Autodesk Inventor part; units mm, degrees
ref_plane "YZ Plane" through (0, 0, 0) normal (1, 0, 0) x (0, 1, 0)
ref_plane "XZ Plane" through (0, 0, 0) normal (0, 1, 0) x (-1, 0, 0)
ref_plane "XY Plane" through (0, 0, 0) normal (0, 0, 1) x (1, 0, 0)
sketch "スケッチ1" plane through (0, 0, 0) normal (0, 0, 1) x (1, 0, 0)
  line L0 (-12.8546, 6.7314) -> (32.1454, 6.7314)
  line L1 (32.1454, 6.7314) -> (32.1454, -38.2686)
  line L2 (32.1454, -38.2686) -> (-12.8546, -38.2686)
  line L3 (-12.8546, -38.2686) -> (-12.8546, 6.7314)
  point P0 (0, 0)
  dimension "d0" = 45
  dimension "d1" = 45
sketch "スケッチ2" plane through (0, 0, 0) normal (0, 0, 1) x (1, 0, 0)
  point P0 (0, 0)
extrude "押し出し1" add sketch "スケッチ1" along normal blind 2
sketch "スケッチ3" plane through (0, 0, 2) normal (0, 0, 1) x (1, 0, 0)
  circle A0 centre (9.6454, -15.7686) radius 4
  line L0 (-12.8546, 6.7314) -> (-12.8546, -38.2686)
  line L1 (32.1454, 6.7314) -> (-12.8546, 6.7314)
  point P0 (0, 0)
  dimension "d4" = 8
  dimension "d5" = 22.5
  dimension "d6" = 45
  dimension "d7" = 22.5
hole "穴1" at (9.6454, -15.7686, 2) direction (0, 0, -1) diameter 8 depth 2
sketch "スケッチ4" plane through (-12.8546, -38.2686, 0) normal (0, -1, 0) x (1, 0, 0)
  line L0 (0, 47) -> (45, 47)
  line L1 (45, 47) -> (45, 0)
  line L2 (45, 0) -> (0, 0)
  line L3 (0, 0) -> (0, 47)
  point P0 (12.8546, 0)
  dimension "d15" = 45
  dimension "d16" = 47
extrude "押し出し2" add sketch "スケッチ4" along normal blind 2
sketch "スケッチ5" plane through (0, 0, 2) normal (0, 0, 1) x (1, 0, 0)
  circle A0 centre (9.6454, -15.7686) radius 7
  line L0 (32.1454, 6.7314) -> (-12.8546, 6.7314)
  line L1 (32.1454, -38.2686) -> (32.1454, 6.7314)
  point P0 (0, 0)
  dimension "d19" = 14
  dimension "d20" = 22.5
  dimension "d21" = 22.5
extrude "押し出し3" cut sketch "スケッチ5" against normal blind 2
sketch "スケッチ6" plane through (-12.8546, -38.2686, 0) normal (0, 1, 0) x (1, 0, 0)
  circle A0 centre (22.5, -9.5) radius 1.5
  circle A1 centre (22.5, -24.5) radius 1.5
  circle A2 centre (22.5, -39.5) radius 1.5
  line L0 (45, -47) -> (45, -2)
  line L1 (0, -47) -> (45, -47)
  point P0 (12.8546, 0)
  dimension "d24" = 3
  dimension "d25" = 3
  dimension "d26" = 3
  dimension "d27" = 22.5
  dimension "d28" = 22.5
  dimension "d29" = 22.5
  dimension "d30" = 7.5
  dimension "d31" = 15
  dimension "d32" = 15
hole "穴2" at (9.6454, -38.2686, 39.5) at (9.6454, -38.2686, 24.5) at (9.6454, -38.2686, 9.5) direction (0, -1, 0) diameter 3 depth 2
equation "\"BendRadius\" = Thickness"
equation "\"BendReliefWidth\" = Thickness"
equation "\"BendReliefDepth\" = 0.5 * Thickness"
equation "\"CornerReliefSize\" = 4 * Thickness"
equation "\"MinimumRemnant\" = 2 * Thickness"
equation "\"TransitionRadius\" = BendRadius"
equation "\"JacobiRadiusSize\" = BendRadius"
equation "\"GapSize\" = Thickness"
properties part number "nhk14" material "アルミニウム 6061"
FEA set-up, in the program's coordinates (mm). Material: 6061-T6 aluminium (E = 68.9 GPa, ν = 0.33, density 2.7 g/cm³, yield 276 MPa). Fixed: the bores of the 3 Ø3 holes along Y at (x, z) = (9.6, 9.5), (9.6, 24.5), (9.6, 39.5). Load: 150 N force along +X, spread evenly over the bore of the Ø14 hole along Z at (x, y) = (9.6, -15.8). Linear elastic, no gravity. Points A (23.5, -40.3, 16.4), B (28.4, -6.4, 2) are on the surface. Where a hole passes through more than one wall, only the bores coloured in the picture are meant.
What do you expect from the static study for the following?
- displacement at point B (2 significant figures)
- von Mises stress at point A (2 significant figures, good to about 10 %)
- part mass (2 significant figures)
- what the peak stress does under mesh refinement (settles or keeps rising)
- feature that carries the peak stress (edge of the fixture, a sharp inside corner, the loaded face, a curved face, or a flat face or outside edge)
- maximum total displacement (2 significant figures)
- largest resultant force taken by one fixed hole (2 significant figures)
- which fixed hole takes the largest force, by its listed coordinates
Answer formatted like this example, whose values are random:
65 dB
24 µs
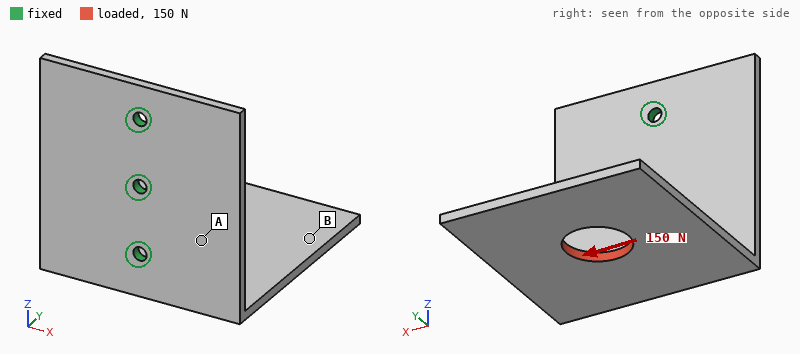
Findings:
0.42 mm
37 MPa
21 g
keeps rising
edge of the fixture
0.57 mm
180 N
(9.6, 9.5)
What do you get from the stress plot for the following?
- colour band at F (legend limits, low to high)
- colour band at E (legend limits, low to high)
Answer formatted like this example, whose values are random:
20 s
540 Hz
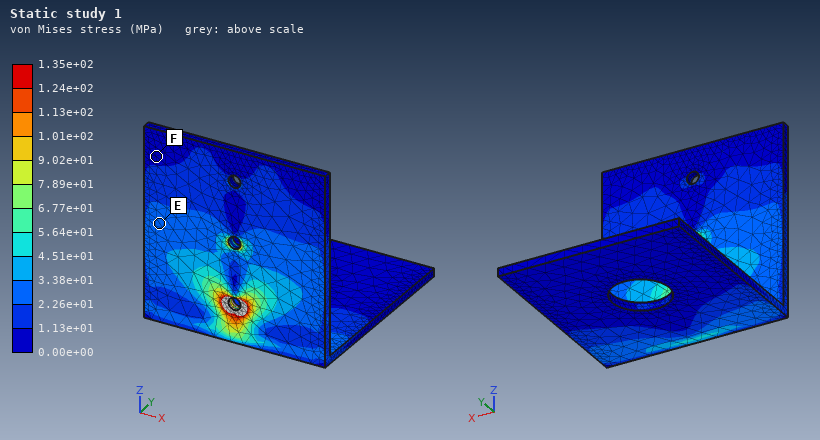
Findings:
0.00e+00 to 1.13e+01 MPa
2.26e+01 to 3.38e+01 MPa
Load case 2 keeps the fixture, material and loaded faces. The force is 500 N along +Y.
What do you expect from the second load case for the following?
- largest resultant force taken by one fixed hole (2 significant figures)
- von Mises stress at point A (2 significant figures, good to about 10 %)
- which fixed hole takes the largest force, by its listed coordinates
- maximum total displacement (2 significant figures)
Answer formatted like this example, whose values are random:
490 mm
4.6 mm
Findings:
600 N
30 MPa
(9.6, 9.5)
0.57 mm
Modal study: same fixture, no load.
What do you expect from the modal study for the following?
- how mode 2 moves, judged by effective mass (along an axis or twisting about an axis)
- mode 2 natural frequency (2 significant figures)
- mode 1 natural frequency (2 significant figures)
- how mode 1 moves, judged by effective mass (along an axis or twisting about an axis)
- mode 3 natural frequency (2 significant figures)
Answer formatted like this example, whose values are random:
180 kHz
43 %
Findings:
along X
910 Hz
580 Hz
along Z
1700 Hz
